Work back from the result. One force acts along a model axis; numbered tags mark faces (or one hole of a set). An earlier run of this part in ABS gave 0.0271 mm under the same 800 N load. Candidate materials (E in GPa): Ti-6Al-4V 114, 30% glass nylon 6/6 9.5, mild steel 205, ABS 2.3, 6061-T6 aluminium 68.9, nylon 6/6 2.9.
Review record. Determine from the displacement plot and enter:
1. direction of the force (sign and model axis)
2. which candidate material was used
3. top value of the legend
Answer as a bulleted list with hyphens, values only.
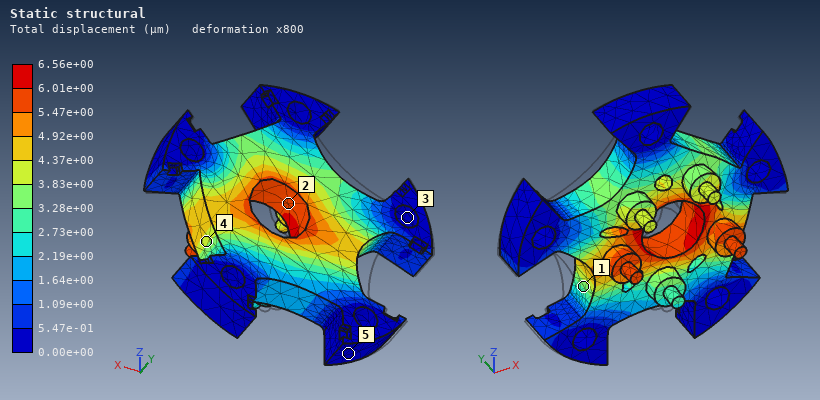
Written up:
- +X
- 30% glass nylon 6/6
- 6.56e+00 µm
